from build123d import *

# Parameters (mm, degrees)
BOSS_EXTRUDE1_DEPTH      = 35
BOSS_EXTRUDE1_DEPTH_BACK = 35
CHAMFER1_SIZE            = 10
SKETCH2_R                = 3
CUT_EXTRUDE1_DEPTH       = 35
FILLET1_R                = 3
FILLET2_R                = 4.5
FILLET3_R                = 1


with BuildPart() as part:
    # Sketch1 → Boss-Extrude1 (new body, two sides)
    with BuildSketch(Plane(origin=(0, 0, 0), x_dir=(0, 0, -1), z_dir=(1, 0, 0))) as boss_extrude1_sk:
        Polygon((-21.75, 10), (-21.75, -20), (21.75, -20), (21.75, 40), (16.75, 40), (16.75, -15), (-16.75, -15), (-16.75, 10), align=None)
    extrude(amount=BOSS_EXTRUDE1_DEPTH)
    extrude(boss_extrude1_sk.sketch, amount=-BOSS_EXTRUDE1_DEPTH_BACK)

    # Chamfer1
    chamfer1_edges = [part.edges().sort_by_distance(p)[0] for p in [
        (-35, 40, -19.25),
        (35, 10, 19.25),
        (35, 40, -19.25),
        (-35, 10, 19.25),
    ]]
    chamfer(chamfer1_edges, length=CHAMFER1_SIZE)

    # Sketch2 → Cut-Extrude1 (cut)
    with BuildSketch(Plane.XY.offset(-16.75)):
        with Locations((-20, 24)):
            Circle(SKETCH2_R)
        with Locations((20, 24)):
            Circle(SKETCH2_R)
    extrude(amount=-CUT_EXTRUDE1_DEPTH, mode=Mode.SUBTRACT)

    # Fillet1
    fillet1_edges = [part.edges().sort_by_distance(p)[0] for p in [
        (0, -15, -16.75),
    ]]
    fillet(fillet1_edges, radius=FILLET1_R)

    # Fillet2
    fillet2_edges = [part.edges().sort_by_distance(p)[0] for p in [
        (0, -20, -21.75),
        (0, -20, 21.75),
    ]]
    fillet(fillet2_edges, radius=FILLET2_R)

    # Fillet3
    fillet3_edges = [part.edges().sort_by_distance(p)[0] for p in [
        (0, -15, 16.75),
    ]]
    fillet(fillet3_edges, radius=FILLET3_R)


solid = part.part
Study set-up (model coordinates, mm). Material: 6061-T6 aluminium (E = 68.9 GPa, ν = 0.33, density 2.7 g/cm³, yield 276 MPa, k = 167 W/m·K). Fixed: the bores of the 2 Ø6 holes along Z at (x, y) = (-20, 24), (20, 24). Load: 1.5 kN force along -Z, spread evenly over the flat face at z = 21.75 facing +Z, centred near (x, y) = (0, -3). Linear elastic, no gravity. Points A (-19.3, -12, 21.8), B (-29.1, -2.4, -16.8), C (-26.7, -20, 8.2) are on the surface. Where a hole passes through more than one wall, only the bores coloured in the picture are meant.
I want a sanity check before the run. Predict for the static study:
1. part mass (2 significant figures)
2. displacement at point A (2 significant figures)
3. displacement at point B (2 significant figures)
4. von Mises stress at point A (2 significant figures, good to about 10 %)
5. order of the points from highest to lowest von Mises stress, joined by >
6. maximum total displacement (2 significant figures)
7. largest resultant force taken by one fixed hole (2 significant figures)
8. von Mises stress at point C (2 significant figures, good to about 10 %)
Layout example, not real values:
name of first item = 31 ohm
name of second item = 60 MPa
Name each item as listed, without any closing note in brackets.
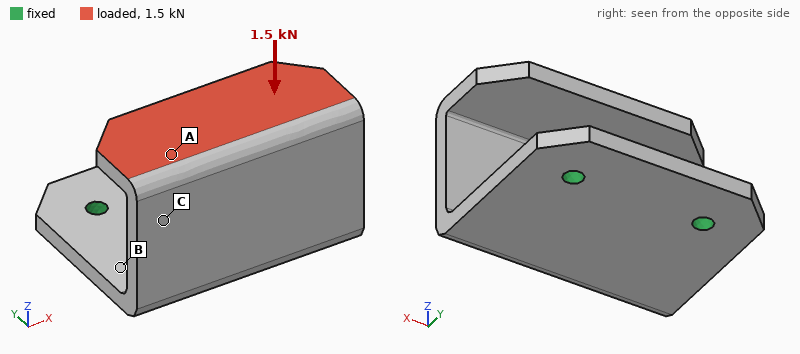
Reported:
part mass = 110 g
displacement at point A = 0.39 mm
displacement at point B = 0.20 mm
von Mises stress at point A = 43 MPa
order of the points from highest to lowest von Mises stress, joined by > = C > A > B
maximum total displacement = 0.56 mm
largest resultant force taken by one fixed hole = 750 N
von Mises stress at point C = 63 MPa
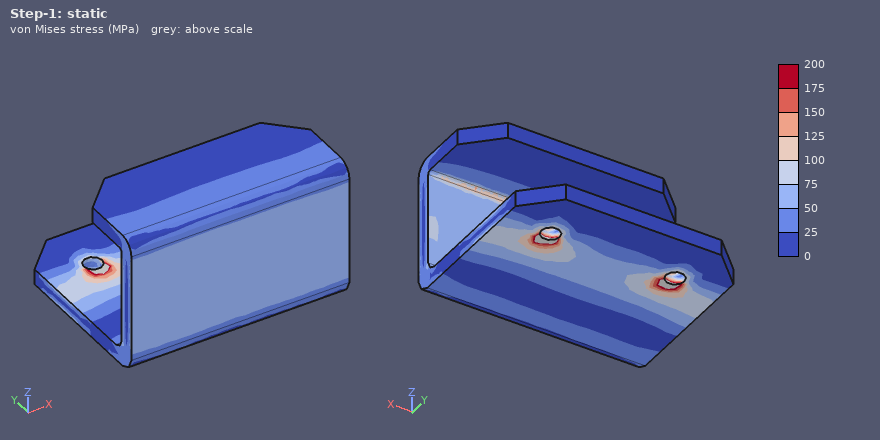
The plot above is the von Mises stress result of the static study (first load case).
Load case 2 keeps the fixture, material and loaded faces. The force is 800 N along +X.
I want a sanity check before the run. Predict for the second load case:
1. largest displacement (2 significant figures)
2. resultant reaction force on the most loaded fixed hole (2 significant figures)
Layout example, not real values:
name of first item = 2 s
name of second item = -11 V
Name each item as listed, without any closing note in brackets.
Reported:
largest displacement = 0.62 mm
resultant reaction force on the most loaded fixed hole = 930 N
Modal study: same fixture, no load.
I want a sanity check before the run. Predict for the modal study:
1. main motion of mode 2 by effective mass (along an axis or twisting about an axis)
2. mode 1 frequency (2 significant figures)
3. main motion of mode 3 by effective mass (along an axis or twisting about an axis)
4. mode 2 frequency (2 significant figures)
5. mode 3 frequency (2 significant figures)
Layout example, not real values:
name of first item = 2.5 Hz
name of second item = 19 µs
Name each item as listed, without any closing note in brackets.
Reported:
main motion of mode 2 by effective mass = along X
mode 1 frequency = 620 Hz
main motion of mode 3 by effective mass = along Z
mode 2 frequency = 1000 Hz
mode 3 frequency = 1400 Hz
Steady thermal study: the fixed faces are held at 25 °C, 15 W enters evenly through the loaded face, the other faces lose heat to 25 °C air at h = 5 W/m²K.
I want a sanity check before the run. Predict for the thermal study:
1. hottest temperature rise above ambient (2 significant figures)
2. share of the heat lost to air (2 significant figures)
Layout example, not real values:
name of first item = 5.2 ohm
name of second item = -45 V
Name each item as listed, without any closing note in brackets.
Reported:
hottest temperature rise above ambient = 23 K
share of the heat lost to air = 5.7 %
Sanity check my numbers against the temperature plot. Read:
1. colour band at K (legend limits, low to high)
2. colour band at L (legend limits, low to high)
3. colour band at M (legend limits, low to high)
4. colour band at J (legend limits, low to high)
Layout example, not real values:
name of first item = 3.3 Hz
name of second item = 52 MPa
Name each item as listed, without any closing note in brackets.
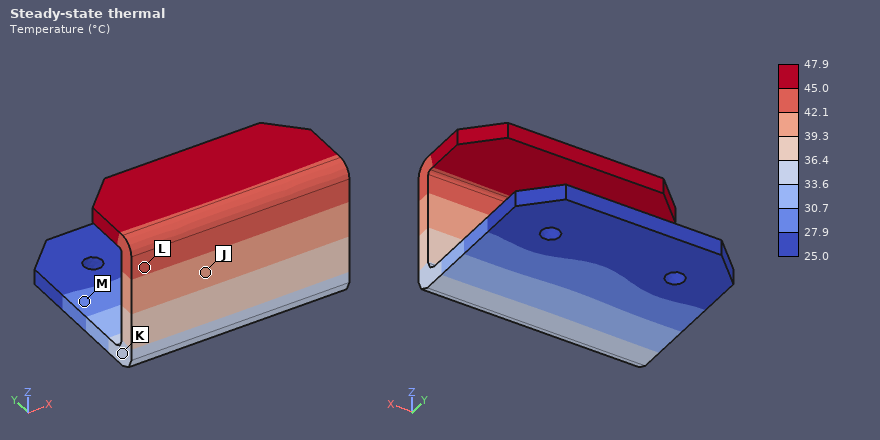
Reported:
colour band at K = 33.6 to 36.4 °C
colour band at L = 42.1 to 45.0 °C
colour band at M = 27.9 to 30.7 °C
colour band at J = 39.3 to 42.1 °C
